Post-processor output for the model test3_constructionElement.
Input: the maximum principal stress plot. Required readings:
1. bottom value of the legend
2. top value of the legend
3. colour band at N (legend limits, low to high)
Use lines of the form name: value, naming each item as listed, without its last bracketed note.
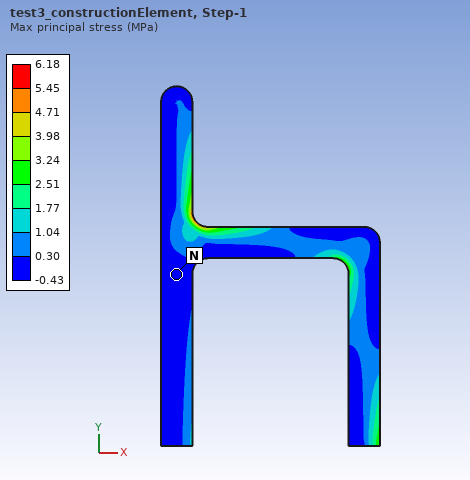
bottom value of the legend: -0.43 MPa
top value of the legend: 6.18 MPa
colour band at N: -0.43 to 0.30 MPa
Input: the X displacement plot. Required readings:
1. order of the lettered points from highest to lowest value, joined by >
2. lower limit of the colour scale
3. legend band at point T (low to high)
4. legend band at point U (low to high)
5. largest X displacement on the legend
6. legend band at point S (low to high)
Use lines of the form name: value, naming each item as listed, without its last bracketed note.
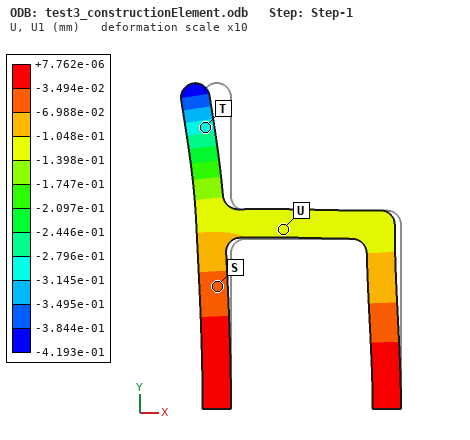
order of the lettered points from highest to lowest value, joined by >: S > U > T
lower limit of the colour scale: -4.193e-01 mm
legend band at point T: -3.145e-01 to -2.796e-01 mm
legend band at point U: -1.398e-01 to -1.048e-01 mm
largest X displacement on the legend: +7.762e-06 mm
legend band at point S: -6.988e-02 to -3.494e-02 mm
